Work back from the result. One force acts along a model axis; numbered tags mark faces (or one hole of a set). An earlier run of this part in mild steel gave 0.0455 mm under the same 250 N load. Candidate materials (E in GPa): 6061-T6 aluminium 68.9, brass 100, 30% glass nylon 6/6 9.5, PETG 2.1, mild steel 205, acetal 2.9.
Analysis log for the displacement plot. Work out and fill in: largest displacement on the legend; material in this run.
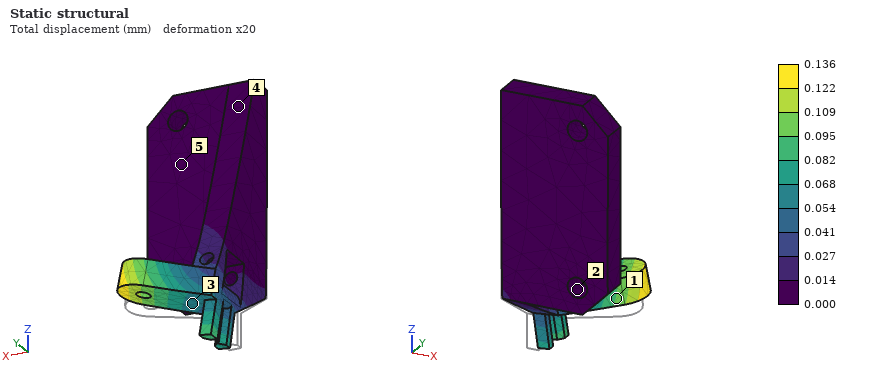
0.136 mm
6061-T6 aluminium
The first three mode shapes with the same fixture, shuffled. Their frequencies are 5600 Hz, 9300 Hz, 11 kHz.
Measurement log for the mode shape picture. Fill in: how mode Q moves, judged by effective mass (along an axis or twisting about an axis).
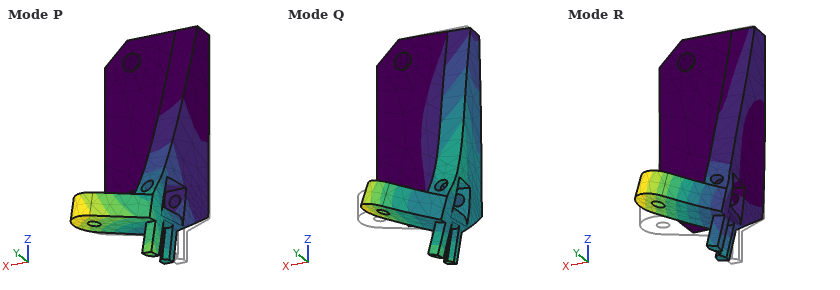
along Y
